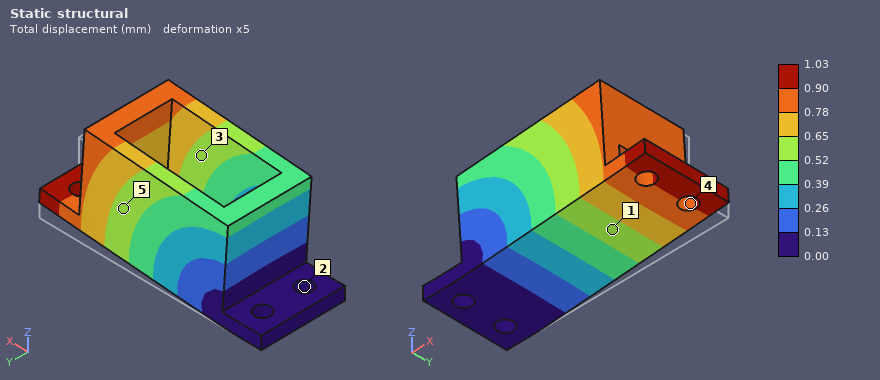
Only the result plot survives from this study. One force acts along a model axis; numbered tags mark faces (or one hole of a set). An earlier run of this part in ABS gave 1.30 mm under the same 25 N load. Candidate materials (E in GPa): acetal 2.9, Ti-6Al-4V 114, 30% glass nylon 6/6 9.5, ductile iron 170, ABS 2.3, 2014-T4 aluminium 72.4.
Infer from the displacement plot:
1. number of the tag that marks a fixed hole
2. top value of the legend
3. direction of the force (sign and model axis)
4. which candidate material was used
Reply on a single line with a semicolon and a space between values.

2; 1.03 mm; +Z; acetal
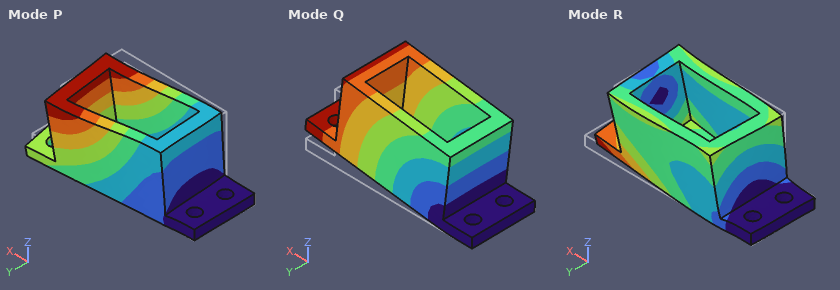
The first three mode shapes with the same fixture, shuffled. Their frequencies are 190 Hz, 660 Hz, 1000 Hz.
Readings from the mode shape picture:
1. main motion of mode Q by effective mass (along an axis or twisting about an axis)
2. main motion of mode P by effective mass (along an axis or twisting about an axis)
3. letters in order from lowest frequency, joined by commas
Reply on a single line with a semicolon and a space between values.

along Z; along Y; Q, P, R
